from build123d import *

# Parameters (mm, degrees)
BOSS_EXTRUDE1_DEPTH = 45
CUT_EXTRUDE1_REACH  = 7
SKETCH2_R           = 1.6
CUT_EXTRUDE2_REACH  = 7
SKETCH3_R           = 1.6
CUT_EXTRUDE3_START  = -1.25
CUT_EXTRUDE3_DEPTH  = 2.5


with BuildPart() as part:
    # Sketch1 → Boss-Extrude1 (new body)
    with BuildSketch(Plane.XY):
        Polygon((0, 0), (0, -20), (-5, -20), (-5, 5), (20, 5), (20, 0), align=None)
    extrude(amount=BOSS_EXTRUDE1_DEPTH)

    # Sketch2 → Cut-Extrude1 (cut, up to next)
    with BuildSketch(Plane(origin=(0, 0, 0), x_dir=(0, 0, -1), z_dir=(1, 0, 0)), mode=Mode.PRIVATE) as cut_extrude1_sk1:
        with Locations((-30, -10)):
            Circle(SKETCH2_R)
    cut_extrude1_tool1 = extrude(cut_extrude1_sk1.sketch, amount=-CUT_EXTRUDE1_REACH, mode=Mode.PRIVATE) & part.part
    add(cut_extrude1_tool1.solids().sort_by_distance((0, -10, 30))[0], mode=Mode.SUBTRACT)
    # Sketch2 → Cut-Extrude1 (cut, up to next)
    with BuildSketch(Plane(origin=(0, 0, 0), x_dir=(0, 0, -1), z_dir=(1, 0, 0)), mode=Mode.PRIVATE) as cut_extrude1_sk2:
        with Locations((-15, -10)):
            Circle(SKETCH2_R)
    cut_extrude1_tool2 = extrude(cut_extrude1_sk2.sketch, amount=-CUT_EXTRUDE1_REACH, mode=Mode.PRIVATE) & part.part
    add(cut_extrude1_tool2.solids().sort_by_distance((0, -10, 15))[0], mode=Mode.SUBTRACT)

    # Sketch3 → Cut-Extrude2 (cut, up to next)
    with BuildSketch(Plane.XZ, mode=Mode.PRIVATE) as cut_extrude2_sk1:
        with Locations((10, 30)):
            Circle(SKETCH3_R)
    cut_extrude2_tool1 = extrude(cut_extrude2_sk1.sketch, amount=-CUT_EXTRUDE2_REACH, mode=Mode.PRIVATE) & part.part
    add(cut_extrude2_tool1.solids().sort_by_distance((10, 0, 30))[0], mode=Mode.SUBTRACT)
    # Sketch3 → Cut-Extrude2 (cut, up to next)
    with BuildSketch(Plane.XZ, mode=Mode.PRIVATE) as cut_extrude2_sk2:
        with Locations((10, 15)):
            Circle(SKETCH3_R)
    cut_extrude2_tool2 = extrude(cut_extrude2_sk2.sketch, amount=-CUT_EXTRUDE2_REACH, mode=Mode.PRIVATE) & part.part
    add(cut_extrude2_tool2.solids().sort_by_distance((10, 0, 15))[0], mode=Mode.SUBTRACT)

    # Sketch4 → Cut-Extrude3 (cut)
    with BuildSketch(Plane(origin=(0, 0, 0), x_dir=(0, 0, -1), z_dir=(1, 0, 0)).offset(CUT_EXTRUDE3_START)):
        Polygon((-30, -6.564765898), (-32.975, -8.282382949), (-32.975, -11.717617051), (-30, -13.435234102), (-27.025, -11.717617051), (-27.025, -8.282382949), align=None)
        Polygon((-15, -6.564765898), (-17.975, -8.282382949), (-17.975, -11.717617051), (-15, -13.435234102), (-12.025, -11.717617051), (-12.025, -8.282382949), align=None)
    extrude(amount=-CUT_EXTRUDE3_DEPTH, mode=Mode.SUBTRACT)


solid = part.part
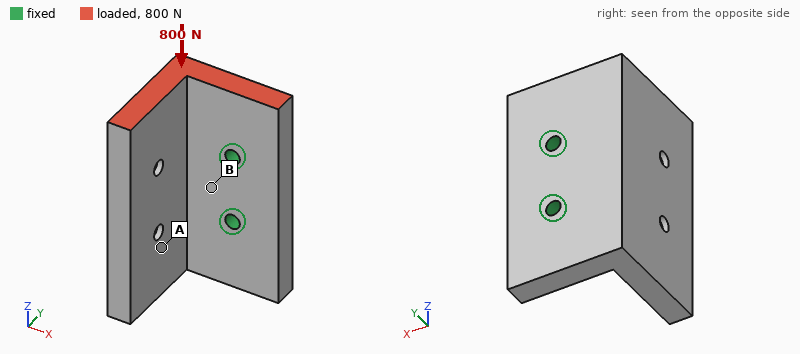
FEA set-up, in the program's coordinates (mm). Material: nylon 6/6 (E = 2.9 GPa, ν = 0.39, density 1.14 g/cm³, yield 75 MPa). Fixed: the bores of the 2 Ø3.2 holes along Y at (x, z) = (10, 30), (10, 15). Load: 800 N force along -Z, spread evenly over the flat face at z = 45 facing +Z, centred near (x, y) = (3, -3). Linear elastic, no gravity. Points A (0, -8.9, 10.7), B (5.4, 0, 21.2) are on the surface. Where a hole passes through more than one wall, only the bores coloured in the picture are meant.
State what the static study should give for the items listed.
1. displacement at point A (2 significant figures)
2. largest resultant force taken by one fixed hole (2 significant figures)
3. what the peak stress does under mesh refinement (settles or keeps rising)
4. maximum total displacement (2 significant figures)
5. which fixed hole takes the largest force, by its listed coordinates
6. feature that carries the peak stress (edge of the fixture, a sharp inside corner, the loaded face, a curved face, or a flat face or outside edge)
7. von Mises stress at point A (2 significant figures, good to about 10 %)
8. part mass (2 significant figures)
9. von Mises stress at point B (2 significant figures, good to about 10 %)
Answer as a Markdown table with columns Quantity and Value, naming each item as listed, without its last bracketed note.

| Quantity | Value |
|---|---|
| displacement at point A | 0.27 mm |
| largest resultant force taken by one fixed hole | 620 N |
| what the peak stress does under mesh refinement | keeps rising |
| maximum total displacement | 0.53 mm |
| which fixed hole takes the largest force, by its listed coordinates | (10, 30) |
| feature that carries the peak stress | edge of the fixture |
| von Mises stress at point A | 6.0 MPa |
| part mass | 11 g |
| von Mises stress at point B | 17 MPa |
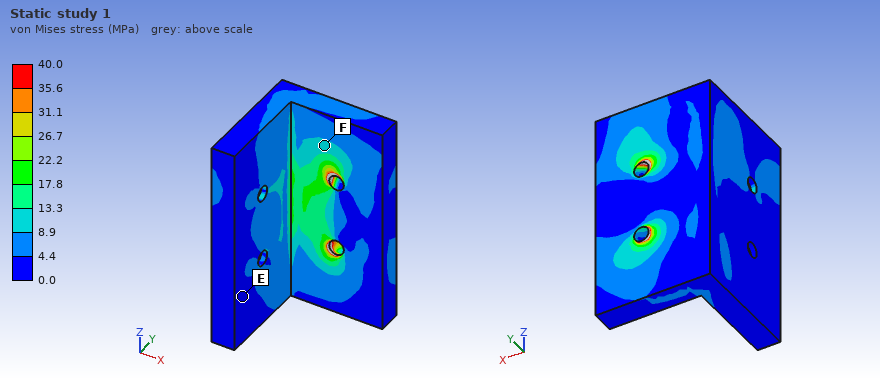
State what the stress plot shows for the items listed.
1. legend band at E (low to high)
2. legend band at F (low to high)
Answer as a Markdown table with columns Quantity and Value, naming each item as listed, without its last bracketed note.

| Quantity | Value |
|---|---|
| legend band at E | 0.0 to 4.4 MPa |
| legend band at F | 8.9 to 13.3 MPa |
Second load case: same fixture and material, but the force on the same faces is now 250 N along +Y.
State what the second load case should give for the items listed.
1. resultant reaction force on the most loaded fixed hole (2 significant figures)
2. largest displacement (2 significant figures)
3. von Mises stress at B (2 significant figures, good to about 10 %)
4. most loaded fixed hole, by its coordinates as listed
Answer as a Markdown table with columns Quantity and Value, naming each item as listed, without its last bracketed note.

| Quantity | Value |
|---|---|
| resultant reaction force on the most loaded fixed hole | 370 N |
| largest displacement | 0.63 mm |
| von Mises stress at B | 8.7 MPa |
| most loaded fixed hole, by its coordinates as listed | (10, 30) |
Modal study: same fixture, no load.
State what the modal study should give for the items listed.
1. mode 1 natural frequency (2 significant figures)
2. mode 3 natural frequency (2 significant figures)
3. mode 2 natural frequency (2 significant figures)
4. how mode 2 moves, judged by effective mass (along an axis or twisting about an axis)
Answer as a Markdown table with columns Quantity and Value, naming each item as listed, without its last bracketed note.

| Quantity | Value |
|---|---|
| mode 1 natural frequency | 1300 Hz |
| mode 3 natural frequency | 3000 Hz |
| mode 2 natural frequency | 1800 Hz |
| how mode 2 moves, judged by effective mass | along Z |
